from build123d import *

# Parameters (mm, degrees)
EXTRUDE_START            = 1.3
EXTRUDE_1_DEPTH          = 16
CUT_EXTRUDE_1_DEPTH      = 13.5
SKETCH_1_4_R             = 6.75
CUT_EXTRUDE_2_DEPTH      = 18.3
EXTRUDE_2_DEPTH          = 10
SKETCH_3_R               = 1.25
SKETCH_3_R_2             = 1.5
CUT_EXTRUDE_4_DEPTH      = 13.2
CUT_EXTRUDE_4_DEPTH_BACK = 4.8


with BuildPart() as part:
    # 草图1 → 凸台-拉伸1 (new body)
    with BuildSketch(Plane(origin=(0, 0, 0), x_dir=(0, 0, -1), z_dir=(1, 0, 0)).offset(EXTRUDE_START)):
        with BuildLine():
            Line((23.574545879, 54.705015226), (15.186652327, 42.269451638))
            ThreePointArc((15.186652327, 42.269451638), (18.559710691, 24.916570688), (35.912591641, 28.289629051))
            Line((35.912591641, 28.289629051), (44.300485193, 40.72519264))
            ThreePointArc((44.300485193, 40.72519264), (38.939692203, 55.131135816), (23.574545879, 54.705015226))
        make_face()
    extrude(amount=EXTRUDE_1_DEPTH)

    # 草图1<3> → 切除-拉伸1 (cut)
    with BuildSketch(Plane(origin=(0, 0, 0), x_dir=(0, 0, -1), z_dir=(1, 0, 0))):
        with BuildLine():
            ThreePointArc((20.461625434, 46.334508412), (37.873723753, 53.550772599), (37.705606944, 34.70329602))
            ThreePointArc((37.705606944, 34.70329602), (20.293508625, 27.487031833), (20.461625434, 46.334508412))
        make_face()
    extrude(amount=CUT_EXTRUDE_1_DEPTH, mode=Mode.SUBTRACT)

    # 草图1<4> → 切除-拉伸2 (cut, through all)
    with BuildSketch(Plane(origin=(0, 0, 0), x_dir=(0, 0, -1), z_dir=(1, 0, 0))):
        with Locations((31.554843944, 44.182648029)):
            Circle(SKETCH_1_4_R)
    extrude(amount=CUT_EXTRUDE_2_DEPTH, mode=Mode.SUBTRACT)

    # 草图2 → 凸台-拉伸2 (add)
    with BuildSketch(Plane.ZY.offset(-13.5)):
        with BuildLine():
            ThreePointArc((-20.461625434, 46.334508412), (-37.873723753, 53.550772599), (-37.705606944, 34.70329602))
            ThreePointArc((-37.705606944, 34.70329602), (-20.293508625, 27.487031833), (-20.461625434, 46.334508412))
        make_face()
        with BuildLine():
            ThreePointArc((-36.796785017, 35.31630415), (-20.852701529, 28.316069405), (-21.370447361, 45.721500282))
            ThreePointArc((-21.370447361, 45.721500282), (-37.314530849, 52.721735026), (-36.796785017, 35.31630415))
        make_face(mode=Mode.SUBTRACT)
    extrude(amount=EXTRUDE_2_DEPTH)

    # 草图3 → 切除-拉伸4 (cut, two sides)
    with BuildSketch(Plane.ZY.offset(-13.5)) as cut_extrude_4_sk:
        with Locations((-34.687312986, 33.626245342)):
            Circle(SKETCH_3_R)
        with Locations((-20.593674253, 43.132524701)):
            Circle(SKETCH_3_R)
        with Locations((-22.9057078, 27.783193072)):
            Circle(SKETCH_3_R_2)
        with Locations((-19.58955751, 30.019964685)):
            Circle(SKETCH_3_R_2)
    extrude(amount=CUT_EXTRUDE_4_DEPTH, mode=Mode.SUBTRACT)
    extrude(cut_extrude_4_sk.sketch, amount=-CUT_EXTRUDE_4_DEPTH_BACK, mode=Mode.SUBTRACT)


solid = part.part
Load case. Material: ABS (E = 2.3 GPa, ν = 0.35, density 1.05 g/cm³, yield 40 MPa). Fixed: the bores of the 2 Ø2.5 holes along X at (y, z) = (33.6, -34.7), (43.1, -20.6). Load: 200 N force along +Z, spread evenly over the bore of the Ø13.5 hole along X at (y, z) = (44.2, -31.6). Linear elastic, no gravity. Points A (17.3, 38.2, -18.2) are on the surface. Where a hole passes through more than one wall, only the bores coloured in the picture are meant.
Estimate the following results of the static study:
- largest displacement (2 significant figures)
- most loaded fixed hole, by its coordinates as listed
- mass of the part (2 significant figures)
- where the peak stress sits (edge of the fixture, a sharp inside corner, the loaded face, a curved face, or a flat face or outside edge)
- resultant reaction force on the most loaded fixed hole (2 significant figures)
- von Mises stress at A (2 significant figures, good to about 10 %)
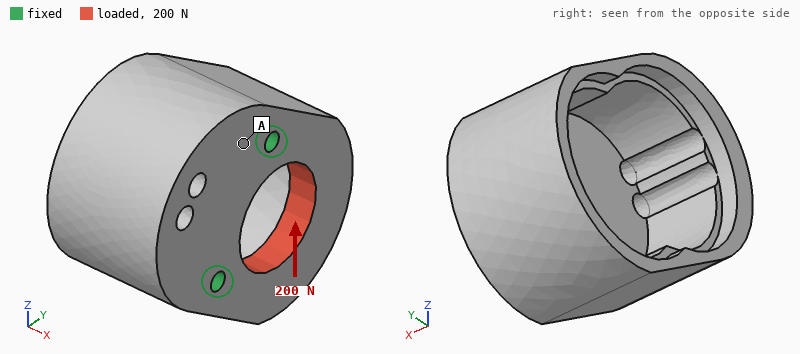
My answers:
87 µm
(43.1, -20.6)
5.7 g
edge of the fixture
140 N
1.5 MPa
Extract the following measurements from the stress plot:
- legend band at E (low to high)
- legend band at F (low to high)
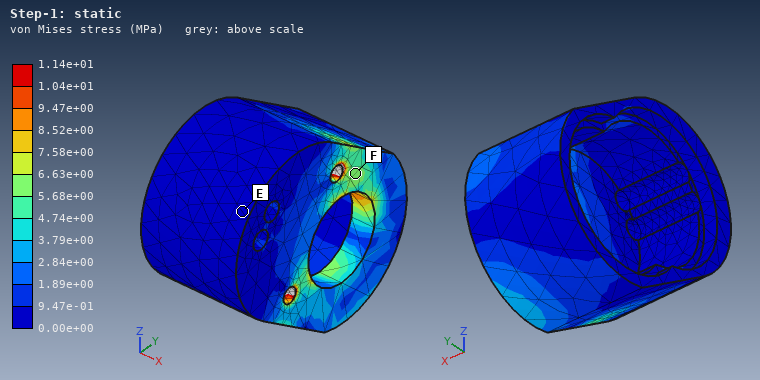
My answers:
0.00e+00 to 9.47e-01 MPa
5.68e+00 to 6.63e+00 MPa
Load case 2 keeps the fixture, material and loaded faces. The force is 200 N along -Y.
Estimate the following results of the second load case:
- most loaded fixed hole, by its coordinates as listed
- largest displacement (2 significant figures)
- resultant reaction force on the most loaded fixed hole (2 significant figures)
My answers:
(33.6, -34.7)
63 µm
130 N
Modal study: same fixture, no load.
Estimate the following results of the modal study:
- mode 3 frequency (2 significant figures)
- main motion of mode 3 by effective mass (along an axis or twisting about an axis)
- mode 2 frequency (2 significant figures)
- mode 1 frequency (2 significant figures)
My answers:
4000 Hz
along X
2900 Hz
1700 Hz
